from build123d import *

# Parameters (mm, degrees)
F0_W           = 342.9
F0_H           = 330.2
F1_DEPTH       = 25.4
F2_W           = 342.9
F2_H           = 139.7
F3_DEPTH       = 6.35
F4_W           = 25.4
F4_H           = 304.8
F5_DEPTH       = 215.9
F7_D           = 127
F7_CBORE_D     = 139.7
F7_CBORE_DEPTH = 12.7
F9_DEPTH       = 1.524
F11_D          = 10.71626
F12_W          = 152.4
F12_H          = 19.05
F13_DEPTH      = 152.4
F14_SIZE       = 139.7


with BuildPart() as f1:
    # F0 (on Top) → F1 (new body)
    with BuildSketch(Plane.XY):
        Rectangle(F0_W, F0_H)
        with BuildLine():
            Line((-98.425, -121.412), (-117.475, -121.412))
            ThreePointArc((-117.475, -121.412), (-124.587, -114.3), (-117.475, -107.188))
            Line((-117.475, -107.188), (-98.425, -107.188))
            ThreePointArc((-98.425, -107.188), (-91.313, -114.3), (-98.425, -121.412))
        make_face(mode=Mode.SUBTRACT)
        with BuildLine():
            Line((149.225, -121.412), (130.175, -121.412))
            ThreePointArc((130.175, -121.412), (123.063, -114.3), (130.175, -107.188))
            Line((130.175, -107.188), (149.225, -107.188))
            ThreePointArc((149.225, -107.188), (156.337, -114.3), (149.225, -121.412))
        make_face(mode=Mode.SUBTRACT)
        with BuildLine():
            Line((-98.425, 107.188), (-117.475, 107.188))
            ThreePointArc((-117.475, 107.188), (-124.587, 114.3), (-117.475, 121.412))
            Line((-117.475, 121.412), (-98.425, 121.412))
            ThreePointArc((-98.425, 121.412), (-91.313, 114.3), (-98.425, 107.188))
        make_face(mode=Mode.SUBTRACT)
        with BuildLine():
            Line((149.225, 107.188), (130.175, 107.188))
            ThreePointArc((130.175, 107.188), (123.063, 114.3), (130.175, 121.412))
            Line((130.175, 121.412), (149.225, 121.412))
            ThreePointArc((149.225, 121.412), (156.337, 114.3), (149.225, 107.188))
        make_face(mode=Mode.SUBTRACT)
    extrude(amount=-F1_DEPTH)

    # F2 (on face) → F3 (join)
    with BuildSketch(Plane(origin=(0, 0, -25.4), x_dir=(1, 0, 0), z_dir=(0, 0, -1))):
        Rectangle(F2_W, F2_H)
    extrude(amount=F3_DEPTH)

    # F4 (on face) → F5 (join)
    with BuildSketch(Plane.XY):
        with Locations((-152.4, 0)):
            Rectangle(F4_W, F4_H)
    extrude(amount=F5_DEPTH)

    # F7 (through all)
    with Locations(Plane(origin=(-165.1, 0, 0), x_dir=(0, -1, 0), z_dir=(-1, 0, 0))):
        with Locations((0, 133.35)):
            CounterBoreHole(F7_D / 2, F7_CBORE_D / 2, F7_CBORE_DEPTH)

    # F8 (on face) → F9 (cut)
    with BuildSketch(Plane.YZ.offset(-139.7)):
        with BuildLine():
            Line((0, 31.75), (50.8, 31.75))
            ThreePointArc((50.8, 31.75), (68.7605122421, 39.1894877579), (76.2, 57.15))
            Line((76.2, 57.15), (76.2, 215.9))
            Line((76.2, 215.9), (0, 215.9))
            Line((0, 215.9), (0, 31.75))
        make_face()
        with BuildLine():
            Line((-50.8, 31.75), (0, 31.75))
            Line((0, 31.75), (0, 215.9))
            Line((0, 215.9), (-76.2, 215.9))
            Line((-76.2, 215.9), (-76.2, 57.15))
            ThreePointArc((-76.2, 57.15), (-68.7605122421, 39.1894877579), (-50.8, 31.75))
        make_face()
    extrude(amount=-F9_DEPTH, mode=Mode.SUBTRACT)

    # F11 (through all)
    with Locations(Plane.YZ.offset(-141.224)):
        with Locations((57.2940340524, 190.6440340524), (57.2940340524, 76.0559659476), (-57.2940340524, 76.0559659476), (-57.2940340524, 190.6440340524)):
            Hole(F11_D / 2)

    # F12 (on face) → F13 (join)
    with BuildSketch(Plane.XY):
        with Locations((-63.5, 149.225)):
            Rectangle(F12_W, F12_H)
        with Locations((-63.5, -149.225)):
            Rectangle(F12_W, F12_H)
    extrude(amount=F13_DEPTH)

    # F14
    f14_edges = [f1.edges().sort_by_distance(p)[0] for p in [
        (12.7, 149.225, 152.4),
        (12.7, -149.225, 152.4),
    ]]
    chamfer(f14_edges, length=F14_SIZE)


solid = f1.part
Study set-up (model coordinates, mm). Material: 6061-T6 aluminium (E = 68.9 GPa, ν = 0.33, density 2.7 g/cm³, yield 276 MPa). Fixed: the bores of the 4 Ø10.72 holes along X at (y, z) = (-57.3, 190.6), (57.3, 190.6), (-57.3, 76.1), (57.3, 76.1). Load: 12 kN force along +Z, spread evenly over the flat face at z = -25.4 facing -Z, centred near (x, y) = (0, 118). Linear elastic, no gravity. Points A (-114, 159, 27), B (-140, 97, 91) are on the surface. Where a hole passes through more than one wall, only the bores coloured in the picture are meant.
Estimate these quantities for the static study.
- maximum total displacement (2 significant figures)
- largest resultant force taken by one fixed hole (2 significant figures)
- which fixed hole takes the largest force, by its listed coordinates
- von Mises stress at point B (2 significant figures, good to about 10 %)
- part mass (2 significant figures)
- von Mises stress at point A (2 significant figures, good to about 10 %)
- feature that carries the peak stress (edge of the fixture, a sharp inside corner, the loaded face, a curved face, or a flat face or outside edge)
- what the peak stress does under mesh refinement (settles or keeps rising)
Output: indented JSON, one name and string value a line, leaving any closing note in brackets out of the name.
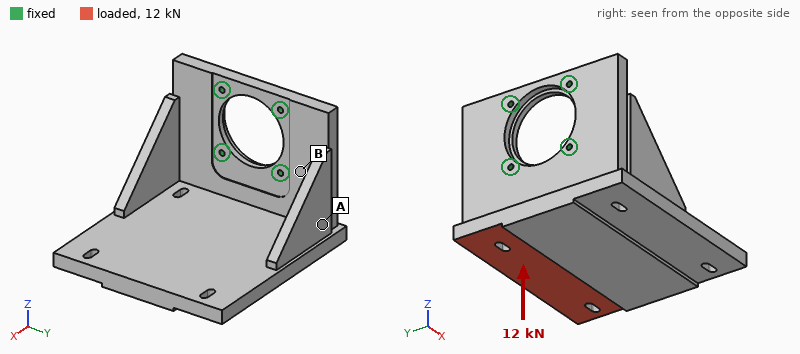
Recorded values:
{
  "maximum total displacement": "1.4 mm",
  "largest resultant force taken by one fixed hole": "13 kN",
  "which fixed hole takes the largest force, by its listed coordinates": "(57.3, 76.1)",
  "von Mises stress at point B": "38 MPa",
  "part mass": "13 kg",
  "von Mises stress at point A": "11 MPa",
  "feature that carries the peak stress": "edge of the fixture",
  "what the peak stress does under mesh refinement": "keeps rising"
}
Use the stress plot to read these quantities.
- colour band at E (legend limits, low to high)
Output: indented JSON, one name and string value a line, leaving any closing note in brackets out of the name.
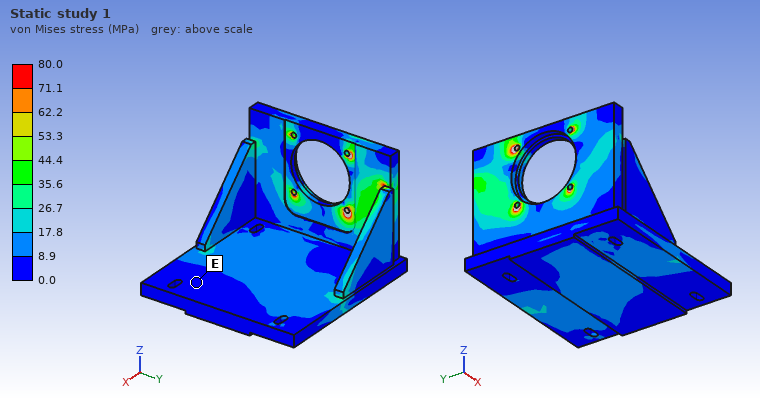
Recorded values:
{
  "colour band at E": "0.0 to 8.9 MPa"
}
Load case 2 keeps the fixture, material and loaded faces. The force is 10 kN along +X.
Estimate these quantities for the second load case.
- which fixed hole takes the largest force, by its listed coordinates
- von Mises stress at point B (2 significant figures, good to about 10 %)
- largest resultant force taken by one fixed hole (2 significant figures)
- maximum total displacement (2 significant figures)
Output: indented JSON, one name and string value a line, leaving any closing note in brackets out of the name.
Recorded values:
{
  "which fixed hole takes the largest force, by its listed coordinates": "(57.3, 76.1)",
  "von Mises stress at point B": "21 MPa",
  "largest resultant force taken by one fixed hole": "15 kN",
  "maximum total displacement": "0.72 mm"
}
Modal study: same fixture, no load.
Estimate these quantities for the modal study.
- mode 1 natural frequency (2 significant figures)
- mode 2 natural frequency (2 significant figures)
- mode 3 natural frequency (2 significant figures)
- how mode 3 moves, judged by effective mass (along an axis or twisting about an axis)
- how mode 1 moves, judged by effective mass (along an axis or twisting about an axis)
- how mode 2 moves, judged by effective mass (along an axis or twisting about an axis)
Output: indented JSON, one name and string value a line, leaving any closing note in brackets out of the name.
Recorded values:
{
  "mode 1 natural frequency": "210 Hz",
  "mode 2 natural frequency": "270 Hz",
  "mode 3 natural frequency": "670 Hz",
  "how mode 3 moves, judged by effective mass": "along X",
  "how mode 1 moves, judged by effective mass": "along Z",
  "how mode 2 moves, judged by effective mass": "along Y"
}
